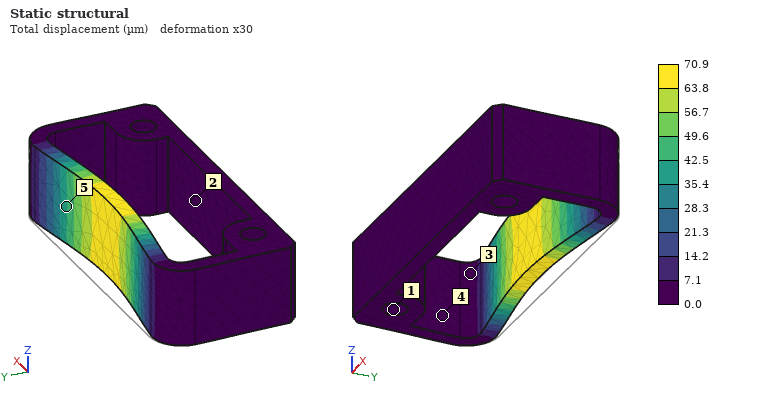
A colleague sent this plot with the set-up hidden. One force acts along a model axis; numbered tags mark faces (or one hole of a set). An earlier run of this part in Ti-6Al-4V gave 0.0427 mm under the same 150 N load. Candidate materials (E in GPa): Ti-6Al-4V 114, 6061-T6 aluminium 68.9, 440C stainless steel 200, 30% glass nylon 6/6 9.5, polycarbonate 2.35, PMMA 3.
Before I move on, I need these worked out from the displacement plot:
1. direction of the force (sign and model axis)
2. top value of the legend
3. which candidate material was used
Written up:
-Y
70.9 µm
6061-T6 aluminium
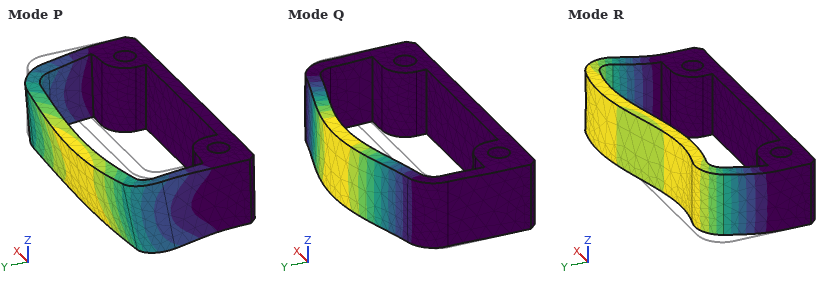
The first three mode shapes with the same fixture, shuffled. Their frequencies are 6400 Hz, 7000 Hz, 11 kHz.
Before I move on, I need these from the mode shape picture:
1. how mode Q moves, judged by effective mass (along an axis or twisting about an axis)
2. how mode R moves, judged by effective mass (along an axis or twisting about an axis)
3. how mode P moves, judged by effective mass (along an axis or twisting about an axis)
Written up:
along Y
along X
along Z
